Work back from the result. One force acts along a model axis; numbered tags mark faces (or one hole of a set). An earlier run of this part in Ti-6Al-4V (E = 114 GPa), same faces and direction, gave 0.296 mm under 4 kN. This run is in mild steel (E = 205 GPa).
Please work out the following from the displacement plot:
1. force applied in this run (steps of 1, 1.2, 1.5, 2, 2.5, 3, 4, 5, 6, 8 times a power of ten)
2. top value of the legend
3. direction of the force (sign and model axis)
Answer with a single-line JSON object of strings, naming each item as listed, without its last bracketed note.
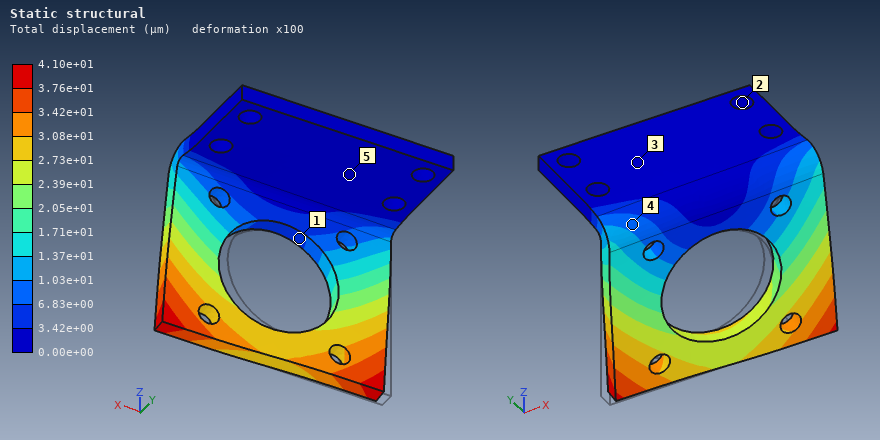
{"force applied in this run": "1 kN", "top value of the legend": "4.10e+01 µm", "direction of the force": "+X"}
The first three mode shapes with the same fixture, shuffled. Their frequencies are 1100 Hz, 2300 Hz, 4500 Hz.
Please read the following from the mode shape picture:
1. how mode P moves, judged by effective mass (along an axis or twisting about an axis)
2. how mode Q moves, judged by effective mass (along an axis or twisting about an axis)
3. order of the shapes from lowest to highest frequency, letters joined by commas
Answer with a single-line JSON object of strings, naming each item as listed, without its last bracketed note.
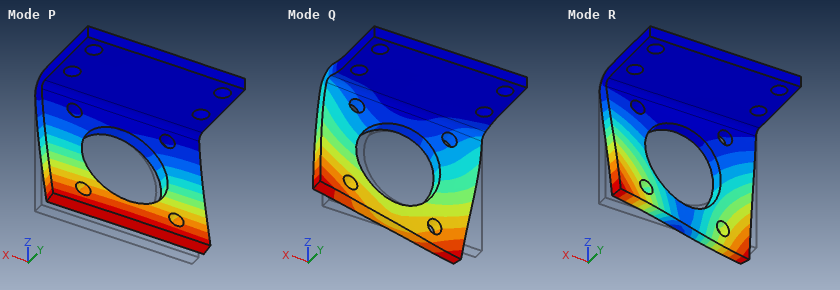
{"how mode P moves, judged by effective mass": "along Y", "how mode Q moves, judged by effective mass": "along X", "order of the shapes from lowest to highest frequency, letters joined by commas": "P, R, Q"}
